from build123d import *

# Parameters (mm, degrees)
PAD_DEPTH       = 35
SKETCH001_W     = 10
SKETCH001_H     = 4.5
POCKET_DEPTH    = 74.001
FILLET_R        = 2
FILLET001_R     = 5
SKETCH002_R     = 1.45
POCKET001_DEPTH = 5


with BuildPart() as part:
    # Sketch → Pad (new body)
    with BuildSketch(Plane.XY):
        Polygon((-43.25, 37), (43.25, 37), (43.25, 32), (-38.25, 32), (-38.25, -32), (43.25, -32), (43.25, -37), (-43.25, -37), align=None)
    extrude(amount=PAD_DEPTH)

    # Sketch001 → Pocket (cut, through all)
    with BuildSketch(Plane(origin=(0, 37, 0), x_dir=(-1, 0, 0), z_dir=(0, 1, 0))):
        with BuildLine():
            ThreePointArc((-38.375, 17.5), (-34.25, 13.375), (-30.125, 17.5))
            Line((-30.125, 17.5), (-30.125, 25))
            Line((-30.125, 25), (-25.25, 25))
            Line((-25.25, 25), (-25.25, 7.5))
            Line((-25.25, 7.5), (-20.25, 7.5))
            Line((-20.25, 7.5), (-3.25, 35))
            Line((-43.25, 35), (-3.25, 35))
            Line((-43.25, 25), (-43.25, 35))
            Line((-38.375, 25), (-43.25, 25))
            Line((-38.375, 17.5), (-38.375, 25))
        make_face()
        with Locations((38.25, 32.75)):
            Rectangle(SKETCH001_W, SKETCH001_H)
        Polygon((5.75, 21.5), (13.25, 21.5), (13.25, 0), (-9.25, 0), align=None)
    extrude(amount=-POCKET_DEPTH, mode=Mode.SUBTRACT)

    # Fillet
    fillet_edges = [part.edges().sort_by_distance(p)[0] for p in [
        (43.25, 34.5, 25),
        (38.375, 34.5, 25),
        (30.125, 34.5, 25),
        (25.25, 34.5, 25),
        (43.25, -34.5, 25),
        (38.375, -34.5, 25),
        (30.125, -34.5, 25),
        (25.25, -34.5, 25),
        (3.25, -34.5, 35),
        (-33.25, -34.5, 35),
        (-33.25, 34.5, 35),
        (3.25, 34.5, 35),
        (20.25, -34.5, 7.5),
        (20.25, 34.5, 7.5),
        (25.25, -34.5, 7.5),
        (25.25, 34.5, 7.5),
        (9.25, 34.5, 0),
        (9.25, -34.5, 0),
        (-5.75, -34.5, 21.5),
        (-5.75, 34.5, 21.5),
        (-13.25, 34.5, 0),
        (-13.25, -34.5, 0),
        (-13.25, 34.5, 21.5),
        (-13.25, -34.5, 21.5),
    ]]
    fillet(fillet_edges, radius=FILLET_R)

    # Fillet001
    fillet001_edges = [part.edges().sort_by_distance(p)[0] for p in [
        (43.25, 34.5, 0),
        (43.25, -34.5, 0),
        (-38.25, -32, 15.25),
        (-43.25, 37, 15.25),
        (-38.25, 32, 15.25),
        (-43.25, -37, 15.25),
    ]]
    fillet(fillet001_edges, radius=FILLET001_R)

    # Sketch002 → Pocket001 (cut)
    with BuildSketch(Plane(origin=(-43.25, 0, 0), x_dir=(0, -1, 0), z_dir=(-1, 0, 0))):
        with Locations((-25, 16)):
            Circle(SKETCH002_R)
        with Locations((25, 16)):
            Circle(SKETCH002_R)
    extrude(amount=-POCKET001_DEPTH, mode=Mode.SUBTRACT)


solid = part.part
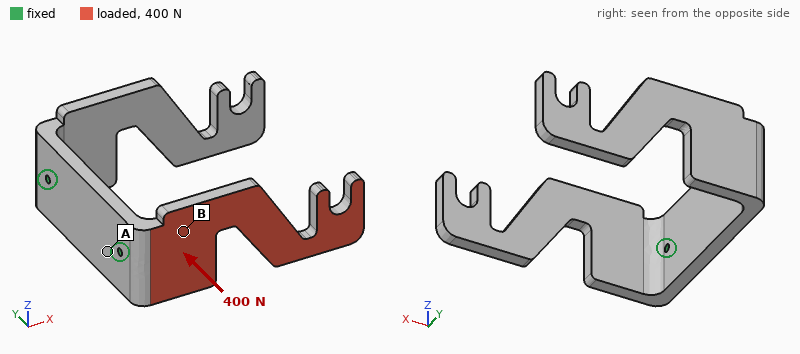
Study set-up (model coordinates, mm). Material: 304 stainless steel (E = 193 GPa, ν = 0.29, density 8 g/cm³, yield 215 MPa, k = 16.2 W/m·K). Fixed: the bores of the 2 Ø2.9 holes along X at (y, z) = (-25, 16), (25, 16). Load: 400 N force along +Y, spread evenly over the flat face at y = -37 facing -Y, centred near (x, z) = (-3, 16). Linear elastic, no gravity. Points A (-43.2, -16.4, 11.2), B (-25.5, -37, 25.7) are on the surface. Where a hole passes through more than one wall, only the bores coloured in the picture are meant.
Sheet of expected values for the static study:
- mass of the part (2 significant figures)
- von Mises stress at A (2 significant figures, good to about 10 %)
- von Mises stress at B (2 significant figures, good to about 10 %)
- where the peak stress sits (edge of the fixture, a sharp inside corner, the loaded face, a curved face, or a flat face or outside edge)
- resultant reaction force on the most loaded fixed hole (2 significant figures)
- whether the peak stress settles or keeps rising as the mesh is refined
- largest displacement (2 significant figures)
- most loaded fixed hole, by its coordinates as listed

240 g
21 MPa
78 MPa
edge of the fixture
400 N
keeps rising
0.75 mm
(-25, 16)
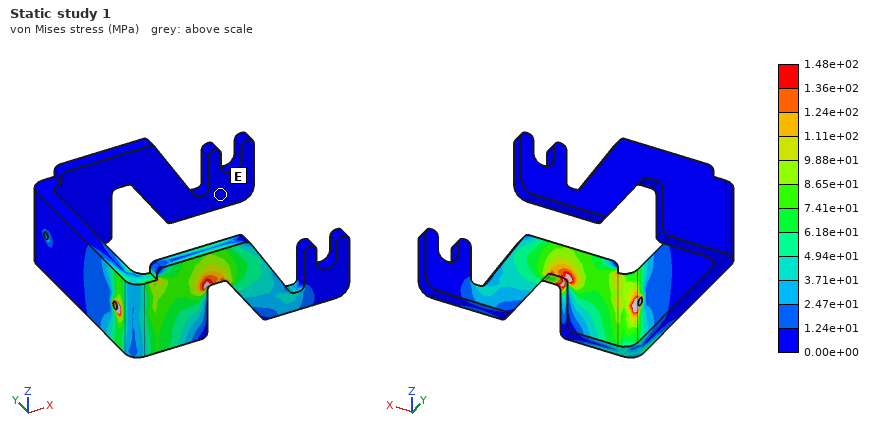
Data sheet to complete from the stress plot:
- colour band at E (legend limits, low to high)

0.00e+00 to 1.24e+01 MPa
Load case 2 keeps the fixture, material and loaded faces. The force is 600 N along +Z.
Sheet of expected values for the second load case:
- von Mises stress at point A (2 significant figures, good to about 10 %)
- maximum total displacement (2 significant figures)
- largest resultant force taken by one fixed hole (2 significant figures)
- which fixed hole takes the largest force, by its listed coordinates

36 MPa
0.30 mm
730 N
(-25, 16)
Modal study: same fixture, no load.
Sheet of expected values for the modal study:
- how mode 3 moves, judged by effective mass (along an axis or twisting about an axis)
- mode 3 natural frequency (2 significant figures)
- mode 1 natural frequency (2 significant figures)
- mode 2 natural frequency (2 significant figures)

along Z
1000 Hz
530 Hz
540 Hz
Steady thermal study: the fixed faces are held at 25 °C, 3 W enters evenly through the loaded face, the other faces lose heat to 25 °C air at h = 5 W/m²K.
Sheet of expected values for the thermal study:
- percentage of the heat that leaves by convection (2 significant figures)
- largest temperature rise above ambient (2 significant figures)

26 %
66 K
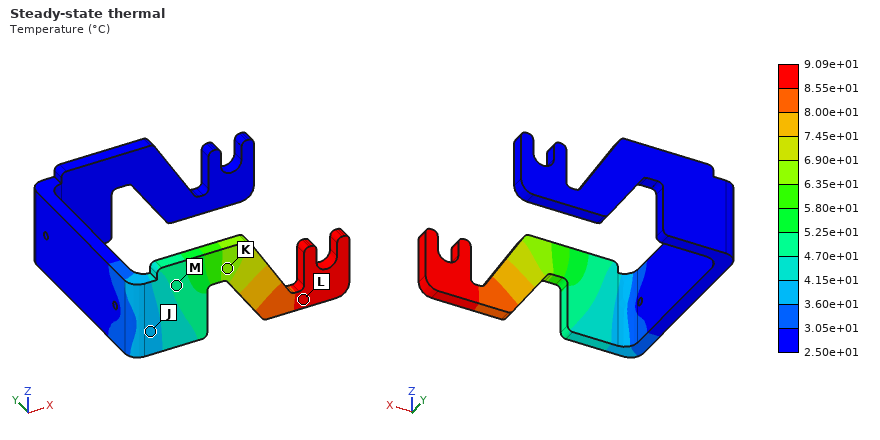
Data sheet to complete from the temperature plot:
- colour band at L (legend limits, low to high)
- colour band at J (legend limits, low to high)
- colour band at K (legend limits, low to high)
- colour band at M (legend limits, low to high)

8.55e+01 to 9.09e+01 °C
3.60e+01 to 4.15e+01 °C
6.35e+01 to 6.90e+01 °C
4.70e+01 to 5.25e+01 °C
